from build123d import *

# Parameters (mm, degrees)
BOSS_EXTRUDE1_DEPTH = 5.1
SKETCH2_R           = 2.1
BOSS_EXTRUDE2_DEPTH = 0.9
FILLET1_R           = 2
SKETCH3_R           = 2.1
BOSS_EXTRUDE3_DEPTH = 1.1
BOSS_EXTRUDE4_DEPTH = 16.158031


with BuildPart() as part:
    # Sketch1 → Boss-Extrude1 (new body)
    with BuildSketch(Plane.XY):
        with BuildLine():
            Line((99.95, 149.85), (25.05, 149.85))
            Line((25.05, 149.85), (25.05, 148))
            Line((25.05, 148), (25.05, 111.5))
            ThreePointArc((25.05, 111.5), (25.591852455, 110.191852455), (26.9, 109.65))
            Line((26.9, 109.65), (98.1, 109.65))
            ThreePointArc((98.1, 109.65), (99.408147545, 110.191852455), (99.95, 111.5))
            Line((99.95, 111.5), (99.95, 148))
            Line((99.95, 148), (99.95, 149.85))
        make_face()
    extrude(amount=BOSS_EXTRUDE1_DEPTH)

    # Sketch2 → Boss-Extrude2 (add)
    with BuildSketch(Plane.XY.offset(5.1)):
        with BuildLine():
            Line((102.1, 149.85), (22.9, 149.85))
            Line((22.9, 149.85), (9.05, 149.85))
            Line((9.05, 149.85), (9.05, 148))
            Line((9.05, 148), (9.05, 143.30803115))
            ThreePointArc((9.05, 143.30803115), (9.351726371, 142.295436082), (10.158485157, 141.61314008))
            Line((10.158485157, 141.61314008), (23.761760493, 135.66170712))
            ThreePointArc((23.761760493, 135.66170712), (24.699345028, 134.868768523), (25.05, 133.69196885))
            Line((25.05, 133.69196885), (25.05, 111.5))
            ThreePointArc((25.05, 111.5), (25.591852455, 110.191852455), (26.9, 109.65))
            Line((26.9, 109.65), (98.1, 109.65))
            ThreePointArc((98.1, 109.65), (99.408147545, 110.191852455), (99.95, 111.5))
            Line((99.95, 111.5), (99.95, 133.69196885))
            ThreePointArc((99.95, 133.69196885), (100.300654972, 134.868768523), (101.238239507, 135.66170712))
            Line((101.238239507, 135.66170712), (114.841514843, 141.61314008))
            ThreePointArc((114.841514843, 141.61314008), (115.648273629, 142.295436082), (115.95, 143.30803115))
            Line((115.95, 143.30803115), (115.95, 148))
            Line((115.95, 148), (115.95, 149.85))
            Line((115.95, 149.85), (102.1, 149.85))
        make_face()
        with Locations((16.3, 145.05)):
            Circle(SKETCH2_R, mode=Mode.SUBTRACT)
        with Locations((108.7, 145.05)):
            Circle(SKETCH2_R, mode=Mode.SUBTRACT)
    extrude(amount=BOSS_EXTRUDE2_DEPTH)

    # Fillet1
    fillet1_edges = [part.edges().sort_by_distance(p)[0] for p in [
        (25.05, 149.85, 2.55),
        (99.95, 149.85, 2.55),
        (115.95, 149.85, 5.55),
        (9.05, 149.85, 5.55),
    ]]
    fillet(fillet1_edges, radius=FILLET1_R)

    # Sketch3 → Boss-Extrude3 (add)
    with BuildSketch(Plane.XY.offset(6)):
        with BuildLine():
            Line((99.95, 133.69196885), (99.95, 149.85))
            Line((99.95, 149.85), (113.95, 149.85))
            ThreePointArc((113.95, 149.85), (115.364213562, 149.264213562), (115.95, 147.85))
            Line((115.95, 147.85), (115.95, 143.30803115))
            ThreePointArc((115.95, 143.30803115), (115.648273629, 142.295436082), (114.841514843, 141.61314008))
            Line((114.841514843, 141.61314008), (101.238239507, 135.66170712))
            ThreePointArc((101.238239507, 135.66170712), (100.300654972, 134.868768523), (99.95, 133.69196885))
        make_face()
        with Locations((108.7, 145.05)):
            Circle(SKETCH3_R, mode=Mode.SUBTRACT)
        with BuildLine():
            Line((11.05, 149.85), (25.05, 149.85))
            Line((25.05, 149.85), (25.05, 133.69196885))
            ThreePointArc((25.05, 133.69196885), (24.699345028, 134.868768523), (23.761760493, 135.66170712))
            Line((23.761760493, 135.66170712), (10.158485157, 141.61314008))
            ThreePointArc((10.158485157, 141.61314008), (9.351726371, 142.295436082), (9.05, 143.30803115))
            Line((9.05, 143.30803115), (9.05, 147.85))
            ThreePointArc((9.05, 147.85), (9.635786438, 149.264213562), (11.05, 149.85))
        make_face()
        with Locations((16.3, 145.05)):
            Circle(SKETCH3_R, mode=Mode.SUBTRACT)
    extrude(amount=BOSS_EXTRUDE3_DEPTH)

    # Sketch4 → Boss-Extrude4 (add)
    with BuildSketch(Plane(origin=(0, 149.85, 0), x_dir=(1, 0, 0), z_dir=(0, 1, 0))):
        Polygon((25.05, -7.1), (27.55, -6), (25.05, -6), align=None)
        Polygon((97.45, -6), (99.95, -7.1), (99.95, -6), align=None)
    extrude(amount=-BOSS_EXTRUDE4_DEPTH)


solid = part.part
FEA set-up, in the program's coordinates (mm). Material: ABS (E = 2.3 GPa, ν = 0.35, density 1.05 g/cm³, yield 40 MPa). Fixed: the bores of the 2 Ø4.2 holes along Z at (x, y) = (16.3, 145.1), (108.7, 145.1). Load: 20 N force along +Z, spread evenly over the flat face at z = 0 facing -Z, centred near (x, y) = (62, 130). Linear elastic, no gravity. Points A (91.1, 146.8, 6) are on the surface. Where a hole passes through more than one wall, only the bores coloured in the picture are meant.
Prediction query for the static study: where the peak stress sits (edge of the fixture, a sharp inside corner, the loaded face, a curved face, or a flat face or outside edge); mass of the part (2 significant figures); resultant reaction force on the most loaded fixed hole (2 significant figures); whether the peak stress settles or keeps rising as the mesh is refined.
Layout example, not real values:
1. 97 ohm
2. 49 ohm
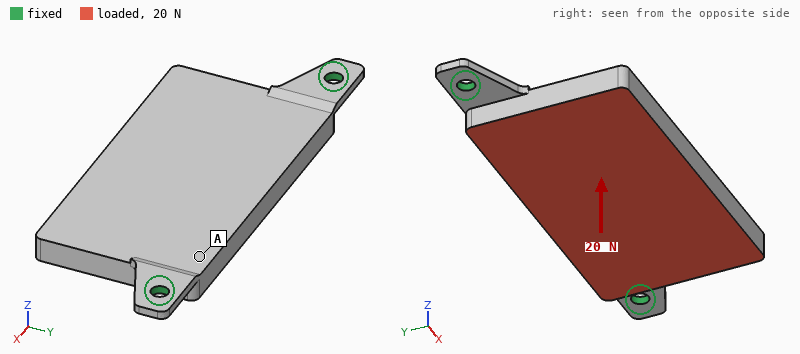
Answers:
1. edge of the fixture
2. 20 g
3. 22 N
4. keeps rising
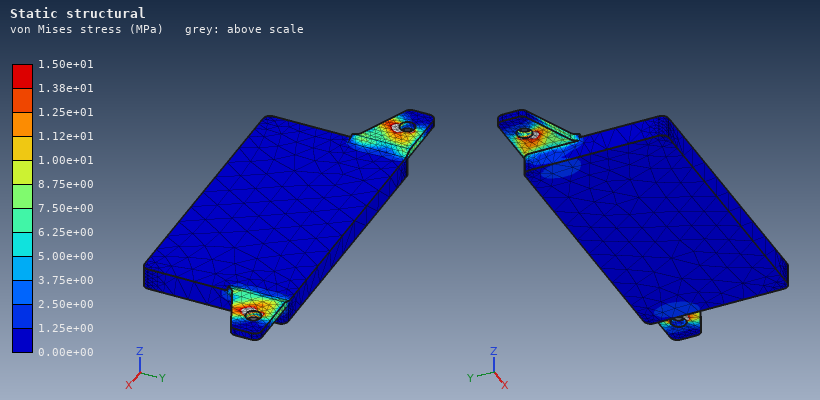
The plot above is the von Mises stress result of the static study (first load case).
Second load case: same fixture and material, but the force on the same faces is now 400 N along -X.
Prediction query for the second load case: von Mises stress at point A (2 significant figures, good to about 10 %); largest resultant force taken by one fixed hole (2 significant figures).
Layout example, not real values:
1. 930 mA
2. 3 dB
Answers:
1. 4.4 MPa
2. 210 N
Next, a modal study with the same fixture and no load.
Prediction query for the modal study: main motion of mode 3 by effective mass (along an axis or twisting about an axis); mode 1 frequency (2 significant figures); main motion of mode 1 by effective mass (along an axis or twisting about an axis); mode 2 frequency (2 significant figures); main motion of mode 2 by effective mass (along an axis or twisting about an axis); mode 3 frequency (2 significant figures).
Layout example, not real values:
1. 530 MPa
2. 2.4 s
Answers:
1. twisting about Y
2. 180 Hz
3. along Z
4. 890 Hz
5. along Z
6. 940 Hz
